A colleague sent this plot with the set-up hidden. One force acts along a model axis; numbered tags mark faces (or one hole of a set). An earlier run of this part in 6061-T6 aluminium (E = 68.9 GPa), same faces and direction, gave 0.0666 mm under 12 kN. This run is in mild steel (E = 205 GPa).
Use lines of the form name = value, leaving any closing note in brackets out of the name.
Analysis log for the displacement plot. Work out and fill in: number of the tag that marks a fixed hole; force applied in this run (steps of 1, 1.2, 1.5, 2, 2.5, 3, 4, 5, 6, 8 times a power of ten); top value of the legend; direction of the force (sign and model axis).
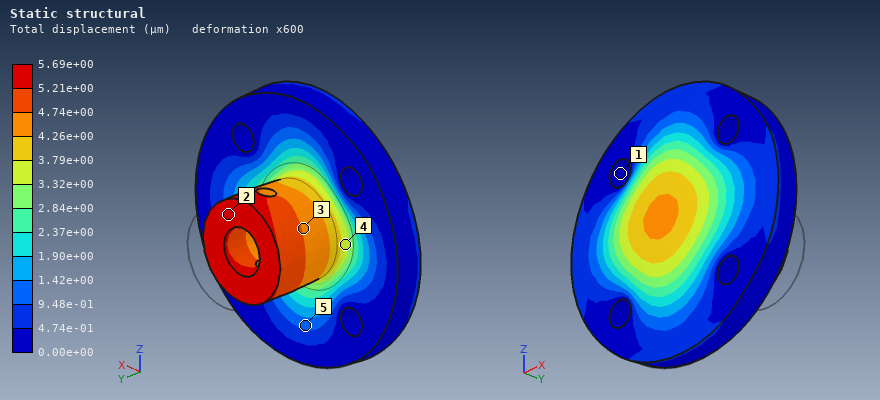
number of the tag that marks a fixed hole = 1
force applied in this run = 3 kN
top value of the legend = 5.69e+00 µm
direction of the force = -Y
